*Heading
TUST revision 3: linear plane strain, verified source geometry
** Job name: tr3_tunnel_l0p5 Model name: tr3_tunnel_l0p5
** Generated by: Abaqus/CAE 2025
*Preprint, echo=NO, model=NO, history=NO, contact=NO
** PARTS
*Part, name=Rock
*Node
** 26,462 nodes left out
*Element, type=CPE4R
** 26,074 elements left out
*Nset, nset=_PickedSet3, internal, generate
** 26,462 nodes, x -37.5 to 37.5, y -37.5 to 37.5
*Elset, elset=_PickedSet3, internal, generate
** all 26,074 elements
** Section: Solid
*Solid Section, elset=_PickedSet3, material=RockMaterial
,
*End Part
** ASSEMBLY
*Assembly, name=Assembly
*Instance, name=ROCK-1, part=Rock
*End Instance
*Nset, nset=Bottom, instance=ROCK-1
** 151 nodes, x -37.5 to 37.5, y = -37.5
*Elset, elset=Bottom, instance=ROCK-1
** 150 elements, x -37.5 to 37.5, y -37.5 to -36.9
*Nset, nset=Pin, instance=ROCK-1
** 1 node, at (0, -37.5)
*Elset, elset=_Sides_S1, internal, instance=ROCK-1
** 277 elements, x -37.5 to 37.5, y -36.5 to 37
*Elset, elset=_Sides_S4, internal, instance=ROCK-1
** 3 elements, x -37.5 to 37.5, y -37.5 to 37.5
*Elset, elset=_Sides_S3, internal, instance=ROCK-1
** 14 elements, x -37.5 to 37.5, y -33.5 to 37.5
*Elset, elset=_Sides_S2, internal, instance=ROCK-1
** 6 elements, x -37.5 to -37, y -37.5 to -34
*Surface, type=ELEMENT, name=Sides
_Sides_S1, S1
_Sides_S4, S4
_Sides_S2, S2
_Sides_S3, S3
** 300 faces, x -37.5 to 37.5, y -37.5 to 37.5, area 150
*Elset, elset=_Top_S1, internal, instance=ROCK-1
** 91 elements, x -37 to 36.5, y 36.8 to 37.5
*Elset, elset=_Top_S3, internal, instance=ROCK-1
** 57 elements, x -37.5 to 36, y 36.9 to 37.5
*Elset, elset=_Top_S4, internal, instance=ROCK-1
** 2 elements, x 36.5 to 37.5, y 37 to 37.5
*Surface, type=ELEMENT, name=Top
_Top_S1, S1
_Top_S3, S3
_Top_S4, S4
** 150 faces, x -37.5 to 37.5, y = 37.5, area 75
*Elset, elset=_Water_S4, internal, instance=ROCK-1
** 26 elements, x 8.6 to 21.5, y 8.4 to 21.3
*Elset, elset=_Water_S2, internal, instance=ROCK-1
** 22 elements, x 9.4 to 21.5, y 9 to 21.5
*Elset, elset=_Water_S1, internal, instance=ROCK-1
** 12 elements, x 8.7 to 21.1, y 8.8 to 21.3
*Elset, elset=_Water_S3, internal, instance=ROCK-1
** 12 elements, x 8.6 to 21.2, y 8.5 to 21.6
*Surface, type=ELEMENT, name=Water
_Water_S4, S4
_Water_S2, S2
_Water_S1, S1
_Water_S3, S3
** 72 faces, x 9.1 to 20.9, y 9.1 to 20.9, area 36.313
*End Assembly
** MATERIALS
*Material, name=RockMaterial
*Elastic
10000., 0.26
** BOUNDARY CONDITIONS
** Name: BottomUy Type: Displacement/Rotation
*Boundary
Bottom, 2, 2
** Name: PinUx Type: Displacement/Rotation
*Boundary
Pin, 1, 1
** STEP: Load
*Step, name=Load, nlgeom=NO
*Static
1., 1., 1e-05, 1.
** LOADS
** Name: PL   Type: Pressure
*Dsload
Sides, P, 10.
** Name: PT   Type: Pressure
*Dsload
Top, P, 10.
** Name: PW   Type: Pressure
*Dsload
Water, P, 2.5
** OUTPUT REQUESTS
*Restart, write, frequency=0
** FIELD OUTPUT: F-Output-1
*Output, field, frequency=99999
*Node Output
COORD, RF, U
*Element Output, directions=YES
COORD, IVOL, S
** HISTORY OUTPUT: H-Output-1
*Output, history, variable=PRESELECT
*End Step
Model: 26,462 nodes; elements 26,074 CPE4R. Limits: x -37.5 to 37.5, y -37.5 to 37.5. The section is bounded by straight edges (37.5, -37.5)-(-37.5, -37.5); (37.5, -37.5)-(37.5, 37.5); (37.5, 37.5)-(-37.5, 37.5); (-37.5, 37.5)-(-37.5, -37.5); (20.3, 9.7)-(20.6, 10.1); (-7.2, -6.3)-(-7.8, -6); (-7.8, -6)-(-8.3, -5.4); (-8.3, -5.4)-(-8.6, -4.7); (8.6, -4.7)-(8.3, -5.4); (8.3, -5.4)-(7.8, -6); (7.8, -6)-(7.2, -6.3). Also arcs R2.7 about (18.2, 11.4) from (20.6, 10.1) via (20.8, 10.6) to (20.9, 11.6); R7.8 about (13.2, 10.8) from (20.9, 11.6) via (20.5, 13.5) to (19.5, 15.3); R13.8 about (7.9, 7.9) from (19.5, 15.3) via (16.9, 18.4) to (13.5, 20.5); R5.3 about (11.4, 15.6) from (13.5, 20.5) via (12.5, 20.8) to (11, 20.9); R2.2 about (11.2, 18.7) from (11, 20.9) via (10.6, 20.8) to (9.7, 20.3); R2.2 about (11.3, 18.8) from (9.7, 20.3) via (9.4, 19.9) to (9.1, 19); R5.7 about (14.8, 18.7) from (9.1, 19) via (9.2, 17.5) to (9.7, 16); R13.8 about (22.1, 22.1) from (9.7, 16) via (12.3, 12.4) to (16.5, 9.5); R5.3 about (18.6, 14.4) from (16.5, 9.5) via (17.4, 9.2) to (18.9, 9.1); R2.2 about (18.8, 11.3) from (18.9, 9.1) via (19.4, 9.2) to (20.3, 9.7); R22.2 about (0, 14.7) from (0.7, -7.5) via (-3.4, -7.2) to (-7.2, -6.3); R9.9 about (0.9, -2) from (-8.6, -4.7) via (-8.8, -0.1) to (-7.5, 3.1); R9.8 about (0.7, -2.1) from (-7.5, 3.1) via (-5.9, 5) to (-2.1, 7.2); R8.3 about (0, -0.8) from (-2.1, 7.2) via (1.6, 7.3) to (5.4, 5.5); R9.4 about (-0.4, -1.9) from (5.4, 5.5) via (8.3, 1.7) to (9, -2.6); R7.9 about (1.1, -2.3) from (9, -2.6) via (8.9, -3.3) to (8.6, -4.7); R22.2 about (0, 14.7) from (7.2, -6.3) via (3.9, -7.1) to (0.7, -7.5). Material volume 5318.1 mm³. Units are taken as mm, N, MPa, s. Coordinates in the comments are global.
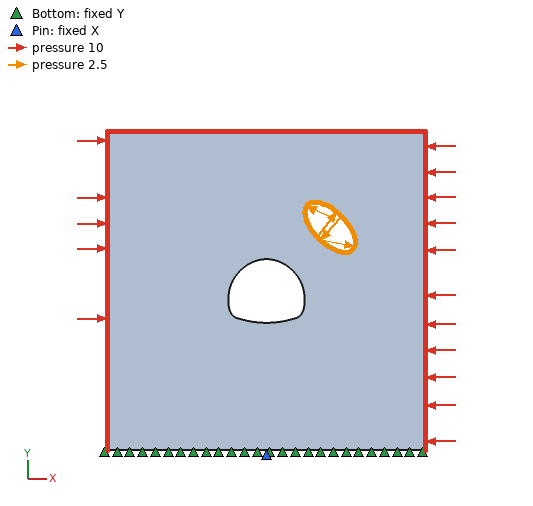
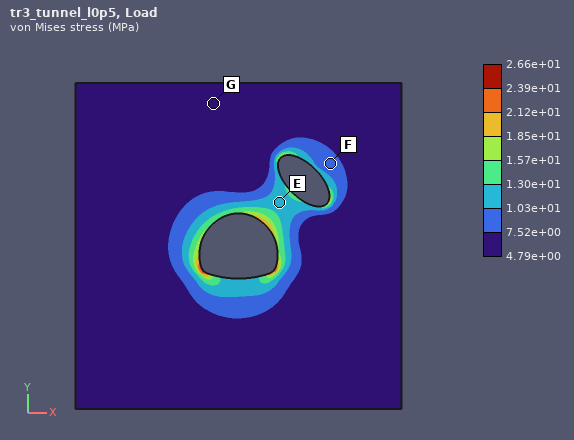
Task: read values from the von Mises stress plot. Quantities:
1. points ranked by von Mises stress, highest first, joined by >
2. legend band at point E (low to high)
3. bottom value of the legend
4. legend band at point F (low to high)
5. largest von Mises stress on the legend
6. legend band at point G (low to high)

E > F > G
1.03e+01 to 1.30e+01 MPa
4.79e+00 MPa
7.52e+00 to 1.03e+01 MPa
2.66e+01 MPa
4.79e+00 to 7.52e+00 MPa
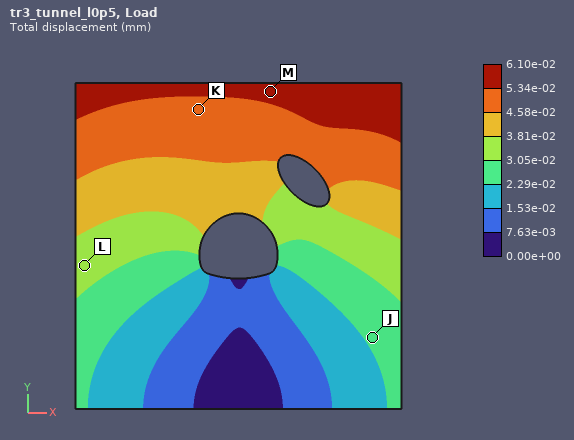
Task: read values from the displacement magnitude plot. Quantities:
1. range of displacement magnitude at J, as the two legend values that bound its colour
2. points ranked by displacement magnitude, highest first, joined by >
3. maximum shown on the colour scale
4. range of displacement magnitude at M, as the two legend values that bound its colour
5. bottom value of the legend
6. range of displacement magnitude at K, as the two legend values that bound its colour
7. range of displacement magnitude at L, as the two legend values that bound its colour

2.29e-02 to 3.05e-02 mm
M > K > L > J
6.10e-02 mm
5.34e-02 to 6.10e-02 mm
0.00e+00 mm
4.58e-02 to 5.34e-02 mm
3.05e-02 to 3.81e-02 mm
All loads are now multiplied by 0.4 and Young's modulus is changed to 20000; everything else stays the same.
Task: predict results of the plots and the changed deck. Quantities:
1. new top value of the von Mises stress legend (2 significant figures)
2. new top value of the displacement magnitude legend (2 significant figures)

11 MPa
0.012 mm
